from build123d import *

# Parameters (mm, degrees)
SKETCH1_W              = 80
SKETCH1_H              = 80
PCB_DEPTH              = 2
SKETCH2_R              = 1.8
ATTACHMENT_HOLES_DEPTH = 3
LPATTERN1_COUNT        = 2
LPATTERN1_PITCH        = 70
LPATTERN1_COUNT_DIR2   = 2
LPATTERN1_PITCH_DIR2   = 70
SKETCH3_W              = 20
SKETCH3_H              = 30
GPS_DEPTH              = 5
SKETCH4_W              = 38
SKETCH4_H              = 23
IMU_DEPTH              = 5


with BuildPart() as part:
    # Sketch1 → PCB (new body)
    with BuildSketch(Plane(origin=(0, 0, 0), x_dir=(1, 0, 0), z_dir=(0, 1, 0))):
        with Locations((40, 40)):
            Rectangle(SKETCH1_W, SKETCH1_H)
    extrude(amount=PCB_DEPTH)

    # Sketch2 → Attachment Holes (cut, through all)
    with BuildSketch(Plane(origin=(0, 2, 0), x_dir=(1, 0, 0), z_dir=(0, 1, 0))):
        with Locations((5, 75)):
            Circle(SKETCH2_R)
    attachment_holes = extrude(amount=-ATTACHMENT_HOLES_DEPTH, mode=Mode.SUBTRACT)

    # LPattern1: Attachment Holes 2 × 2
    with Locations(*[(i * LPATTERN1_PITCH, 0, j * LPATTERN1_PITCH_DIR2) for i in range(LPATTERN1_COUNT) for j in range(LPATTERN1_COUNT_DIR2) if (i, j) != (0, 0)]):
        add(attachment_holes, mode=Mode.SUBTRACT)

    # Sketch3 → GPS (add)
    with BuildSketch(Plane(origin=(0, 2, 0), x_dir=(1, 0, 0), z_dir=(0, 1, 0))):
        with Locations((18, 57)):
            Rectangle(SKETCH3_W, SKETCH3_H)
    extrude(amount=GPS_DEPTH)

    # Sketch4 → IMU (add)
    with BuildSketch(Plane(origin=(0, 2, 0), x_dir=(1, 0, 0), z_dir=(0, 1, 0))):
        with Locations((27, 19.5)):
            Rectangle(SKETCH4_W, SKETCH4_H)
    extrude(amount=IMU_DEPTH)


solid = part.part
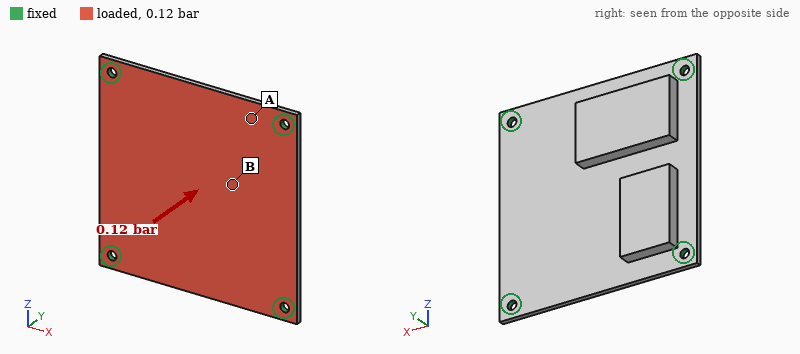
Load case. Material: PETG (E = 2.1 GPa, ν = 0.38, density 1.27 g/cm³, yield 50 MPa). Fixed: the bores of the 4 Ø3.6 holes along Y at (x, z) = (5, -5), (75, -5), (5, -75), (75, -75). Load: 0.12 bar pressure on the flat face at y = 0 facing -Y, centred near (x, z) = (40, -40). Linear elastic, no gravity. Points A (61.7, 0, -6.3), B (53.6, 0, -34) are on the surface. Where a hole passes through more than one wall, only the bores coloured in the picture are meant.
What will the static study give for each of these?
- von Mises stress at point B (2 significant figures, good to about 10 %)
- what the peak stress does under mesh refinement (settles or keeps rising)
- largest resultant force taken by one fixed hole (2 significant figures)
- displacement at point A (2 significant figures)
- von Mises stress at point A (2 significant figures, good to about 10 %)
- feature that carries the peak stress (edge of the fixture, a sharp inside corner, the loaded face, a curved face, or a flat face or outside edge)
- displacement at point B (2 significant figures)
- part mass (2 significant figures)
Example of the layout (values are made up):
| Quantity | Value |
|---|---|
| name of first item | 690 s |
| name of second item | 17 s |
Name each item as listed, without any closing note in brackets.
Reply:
| Quantity | Value |
|---|---|
| von Mises stress at point B | 5.1 MPa |
| what the peak stress does under mesh refinement | keeps rising |
| largest resultant force taken by one fixed hole | 23 N |
| displacement at point A | 0.29 mm |
| von Mises stress at point A | 1.9 MPa |
| feature that carries the peak stress | edge of the fixture |
| displacement at point B | 1.1 mm |
| part mass | 26 g |
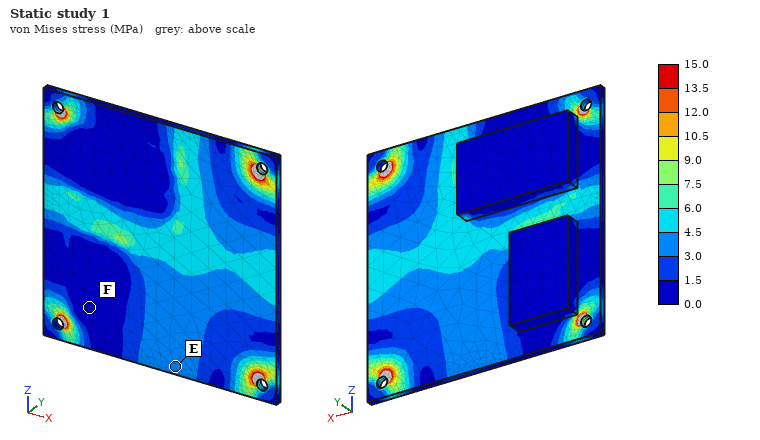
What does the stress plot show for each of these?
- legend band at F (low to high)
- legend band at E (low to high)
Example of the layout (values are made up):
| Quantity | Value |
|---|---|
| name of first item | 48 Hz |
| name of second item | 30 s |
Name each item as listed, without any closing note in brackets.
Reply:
| Quantity | Value |
|---|---|
| legend band at F | 0.0 to 1.5 MPa |
| legend band at E | 3.0 to 4.5 MPa |
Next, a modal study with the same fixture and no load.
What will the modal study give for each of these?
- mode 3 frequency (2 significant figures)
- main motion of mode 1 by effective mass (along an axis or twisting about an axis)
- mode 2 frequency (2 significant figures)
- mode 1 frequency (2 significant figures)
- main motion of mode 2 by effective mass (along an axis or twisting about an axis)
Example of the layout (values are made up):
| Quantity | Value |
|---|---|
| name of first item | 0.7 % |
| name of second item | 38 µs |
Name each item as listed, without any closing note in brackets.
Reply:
| Quantity | Value |
|---|---|
| mode 3 frequency | 730 Hz |
| main motion of mode 1 by effective mass | along Y |
| mode 2 frequency | 650 Hz |
| mode 1 frequency | 330 Hz |
| main motion of mode 2 by effective mass | twisting about Z |
